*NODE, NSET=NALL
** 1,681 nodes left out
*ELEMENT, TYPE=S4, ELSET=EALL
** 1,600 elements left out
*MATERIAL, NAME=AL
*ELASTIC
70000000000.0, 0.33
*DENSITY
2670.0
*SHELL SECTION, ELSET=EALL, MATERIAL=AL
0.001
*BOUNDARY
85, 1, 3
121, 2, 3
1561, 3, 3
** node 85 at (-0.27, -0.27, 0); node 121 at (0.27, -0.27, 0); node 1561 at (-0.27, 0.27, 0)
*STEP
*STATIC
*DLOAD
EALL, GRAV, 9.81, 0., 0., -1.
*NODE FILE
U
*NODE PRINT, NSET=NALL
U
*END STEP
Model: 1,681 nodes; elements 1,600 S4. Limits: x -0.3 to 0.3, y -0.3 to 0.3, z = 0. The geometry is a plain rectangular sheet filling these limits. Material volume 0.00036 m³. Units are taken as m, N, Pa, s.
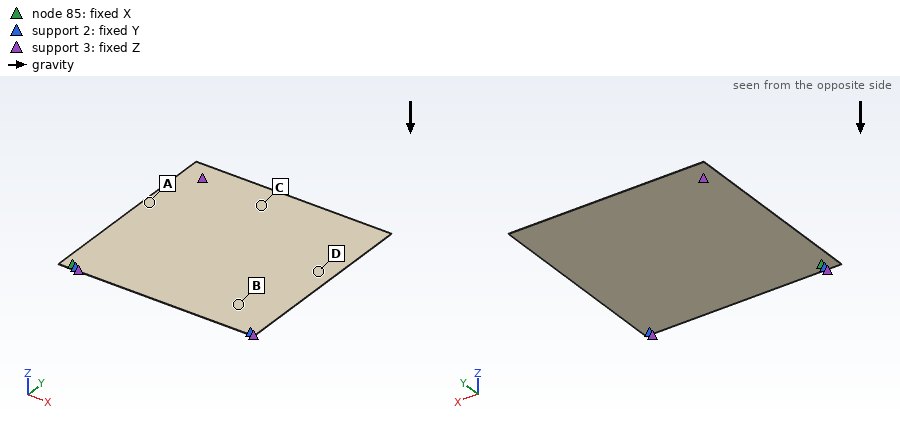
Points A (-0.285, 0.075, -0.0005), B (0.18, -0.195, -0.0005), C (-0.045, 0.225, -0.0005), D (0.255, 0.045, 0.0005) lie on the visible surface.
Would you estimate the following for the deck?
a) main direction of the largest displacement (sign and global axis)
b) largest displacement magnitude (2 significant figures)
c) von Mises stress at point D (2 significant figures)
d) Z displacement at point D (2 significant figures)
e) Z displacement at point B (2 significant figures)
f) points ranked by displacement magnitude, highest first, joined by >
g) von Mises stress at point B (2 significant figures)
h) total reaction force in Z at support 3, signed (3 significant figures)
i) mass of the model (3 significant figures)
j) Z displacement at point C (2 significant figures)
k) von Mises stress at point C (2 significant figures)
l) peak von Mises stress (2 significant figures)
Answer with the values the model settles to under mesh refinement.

-Z
0.070 m
1.1e+07 Pa
-0.042 m
-0.011 m
D > C > B > A
1.3e+07 Pa
9.43 N
0.961 kg
-0.030 m
1.2e+07 Pa
1.4e+07 Pa
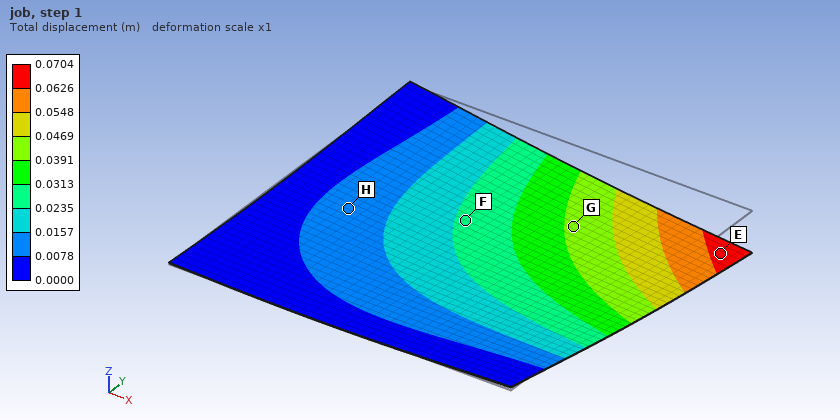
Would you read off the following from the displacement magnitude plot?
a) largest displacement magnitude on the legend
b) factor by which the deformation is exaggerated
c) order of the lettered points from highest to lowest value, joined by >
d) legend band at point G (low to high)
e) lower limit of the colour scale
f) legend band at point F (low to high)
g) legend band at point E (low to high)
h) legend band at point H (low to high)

0.0704 m
1
E > G > F > H
0.0391 to 0.0469 m
0.0000 m
0.0235 to 0.0313 m
0.0626 to 0.0704 m
0.0078 to 0.0157 m
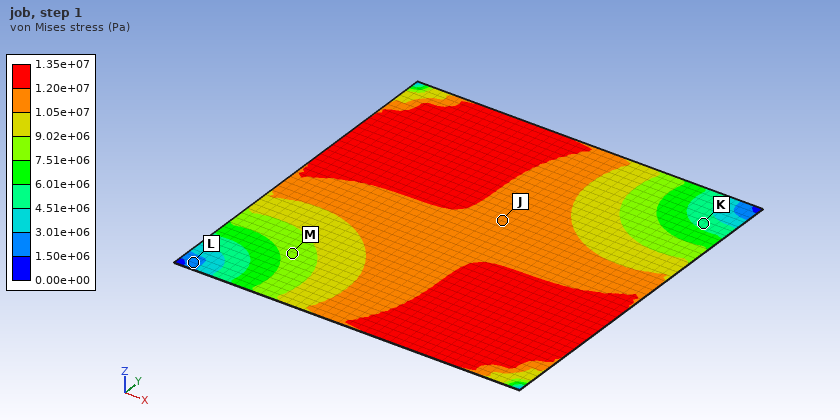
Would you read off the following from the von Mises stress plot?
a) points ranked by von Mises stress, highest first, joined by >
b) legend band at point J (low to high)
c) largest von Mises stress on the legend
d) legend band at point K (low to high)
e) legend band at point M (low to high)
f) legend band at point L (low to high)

J > M > K > L
1.05e+07 to 1.20e+07 Pa
1.35e+07 Pa
4.51e+06 to 6.01e+06 Pa
7.51e+06 to 9.02e+06 Pa
1.50e+06 to 3.01e+06 Pa
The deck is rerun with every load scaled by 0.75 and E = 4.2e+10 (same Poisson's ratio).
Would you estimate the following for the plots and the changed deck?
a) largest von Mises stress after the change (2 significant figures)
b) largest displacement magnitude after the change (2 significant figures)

1.0e+07 Pa
0.088 m
